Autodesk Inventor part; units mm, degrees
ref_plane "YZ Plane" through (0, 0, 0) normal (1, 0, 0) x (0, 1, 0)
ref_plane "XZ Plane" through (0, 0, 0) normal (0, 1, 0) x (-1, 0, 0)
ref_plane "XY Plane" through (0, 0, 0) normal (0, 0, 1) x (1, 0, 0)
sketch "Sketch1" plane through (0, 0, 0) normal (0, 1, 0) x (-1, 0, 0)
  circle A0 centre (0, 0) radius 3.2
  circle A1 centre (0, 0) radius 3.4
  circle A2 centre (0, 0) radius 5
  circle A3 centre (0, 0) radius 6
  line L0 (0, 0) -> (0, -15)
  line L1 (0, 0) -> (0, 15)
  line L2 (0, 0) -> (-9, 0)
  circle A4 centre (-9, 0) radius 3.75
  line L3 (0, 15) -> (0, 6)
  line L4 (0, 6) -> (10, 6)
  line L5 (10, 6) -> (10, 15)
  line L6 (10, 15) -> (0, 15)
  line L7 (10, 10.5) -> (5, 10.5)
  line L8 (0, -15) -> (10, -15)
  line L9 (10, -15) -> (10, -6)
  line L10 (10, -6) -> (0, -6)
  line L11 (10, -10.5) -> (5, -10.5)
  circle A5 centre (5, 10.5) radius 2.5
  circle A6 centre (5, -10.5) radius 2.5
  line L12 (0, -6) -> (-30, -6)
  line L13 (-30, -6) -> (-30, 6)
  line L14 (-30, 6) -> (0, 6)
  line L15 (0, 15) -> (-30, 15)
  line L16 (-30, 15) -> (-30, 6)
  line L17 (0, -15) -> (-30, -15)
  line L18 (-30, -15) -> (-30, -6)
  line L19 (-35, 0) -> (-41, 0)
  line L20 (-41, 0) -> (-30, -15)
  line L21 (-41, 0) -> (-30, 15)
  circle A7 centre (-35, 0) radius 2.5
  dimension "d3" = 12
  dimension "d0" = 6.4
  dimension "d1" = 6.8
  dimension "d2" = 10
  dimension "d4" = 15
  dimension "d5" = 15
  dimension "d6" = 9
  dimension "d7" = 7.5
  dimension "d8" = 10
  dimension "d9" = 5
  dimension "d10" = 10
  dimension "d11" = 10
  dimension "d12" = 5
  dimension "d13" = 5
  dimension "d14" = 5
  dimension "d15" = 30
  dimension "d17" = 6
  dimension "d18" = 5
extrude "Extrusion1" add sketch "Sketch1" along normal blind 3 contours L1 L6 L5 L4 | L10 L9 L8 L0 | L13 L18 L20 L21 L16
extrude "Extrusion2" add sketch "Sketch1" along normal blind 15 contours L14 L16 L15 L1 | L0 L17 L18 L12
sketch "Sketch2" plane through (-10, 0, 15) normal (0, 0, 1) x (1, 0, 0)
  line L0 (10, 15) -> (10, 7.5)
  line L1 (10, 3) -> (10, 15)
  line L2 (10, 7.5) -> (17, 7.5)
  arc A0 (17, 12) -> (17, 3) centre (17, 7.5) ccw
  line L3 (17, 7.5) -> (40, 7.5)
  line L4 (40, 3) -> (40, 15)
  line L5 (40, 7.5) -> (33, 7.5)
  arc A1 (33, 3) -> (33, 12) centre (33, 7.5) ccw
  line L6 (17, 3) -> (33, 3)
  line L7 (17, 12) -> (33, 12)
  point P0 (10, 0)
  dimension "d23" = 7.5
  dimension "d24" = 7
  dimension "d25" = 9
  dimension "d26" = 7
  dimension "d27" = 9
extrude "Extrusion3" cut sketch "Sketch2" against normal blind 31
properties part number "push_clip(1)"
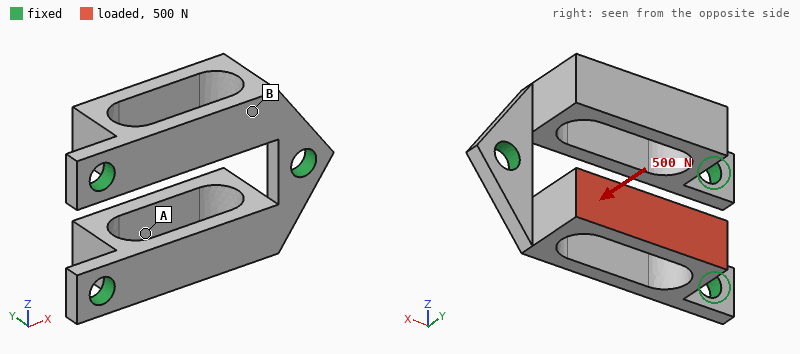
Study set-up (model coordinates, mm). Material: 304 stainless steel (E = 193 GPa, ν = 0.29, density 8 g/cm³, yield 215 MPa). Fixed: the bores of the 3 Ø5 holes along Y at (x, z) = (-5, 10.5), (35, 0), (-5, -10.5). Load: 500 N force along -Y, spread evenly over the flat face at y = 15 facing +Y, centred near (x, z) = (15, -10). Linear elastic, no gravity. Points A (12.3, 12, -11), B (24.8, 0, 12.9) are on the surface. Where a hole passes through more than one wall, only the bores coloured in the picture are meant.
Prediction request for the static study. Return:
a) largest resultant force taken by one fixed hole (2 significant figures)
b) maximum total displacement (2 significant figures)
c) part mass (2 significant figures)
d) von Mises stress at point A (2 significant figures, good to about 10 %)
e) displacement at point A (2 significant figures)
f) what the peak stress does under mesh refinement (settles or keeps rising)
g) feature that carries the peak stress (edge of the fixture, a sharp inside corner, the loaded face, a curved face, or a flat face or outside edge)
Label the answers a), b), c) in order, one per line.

a) 270 N
b) 24 µm
c) 42 g
d) 27 MPa
e) 15 µm
f) keeps rising
g) edge of the fixture
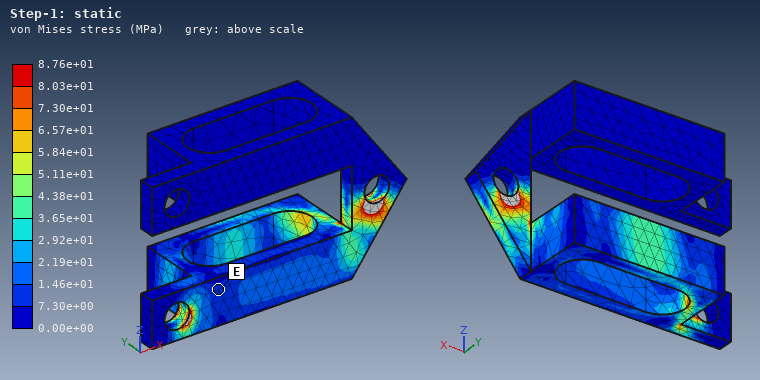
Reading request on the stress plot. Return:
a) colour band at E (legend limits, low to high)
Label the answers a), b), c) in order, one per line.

a) 7.30e+00 to 1.46e+01 MPa
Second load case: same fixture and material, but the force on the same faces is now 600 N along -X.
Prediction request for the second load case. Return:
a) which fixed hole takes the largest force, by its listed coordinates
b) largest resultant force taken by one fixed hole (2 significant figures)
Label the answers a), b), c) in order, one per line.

a) (-5, -10.5)
b) 510 N
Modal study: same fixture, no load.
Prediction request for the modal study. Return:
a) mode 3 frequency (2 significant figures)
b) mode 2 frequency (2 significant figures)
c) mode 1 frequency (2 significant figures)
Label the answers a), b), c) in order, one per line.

a) 10 kHz
b) 5000 Hz
c) 5000 Hz
